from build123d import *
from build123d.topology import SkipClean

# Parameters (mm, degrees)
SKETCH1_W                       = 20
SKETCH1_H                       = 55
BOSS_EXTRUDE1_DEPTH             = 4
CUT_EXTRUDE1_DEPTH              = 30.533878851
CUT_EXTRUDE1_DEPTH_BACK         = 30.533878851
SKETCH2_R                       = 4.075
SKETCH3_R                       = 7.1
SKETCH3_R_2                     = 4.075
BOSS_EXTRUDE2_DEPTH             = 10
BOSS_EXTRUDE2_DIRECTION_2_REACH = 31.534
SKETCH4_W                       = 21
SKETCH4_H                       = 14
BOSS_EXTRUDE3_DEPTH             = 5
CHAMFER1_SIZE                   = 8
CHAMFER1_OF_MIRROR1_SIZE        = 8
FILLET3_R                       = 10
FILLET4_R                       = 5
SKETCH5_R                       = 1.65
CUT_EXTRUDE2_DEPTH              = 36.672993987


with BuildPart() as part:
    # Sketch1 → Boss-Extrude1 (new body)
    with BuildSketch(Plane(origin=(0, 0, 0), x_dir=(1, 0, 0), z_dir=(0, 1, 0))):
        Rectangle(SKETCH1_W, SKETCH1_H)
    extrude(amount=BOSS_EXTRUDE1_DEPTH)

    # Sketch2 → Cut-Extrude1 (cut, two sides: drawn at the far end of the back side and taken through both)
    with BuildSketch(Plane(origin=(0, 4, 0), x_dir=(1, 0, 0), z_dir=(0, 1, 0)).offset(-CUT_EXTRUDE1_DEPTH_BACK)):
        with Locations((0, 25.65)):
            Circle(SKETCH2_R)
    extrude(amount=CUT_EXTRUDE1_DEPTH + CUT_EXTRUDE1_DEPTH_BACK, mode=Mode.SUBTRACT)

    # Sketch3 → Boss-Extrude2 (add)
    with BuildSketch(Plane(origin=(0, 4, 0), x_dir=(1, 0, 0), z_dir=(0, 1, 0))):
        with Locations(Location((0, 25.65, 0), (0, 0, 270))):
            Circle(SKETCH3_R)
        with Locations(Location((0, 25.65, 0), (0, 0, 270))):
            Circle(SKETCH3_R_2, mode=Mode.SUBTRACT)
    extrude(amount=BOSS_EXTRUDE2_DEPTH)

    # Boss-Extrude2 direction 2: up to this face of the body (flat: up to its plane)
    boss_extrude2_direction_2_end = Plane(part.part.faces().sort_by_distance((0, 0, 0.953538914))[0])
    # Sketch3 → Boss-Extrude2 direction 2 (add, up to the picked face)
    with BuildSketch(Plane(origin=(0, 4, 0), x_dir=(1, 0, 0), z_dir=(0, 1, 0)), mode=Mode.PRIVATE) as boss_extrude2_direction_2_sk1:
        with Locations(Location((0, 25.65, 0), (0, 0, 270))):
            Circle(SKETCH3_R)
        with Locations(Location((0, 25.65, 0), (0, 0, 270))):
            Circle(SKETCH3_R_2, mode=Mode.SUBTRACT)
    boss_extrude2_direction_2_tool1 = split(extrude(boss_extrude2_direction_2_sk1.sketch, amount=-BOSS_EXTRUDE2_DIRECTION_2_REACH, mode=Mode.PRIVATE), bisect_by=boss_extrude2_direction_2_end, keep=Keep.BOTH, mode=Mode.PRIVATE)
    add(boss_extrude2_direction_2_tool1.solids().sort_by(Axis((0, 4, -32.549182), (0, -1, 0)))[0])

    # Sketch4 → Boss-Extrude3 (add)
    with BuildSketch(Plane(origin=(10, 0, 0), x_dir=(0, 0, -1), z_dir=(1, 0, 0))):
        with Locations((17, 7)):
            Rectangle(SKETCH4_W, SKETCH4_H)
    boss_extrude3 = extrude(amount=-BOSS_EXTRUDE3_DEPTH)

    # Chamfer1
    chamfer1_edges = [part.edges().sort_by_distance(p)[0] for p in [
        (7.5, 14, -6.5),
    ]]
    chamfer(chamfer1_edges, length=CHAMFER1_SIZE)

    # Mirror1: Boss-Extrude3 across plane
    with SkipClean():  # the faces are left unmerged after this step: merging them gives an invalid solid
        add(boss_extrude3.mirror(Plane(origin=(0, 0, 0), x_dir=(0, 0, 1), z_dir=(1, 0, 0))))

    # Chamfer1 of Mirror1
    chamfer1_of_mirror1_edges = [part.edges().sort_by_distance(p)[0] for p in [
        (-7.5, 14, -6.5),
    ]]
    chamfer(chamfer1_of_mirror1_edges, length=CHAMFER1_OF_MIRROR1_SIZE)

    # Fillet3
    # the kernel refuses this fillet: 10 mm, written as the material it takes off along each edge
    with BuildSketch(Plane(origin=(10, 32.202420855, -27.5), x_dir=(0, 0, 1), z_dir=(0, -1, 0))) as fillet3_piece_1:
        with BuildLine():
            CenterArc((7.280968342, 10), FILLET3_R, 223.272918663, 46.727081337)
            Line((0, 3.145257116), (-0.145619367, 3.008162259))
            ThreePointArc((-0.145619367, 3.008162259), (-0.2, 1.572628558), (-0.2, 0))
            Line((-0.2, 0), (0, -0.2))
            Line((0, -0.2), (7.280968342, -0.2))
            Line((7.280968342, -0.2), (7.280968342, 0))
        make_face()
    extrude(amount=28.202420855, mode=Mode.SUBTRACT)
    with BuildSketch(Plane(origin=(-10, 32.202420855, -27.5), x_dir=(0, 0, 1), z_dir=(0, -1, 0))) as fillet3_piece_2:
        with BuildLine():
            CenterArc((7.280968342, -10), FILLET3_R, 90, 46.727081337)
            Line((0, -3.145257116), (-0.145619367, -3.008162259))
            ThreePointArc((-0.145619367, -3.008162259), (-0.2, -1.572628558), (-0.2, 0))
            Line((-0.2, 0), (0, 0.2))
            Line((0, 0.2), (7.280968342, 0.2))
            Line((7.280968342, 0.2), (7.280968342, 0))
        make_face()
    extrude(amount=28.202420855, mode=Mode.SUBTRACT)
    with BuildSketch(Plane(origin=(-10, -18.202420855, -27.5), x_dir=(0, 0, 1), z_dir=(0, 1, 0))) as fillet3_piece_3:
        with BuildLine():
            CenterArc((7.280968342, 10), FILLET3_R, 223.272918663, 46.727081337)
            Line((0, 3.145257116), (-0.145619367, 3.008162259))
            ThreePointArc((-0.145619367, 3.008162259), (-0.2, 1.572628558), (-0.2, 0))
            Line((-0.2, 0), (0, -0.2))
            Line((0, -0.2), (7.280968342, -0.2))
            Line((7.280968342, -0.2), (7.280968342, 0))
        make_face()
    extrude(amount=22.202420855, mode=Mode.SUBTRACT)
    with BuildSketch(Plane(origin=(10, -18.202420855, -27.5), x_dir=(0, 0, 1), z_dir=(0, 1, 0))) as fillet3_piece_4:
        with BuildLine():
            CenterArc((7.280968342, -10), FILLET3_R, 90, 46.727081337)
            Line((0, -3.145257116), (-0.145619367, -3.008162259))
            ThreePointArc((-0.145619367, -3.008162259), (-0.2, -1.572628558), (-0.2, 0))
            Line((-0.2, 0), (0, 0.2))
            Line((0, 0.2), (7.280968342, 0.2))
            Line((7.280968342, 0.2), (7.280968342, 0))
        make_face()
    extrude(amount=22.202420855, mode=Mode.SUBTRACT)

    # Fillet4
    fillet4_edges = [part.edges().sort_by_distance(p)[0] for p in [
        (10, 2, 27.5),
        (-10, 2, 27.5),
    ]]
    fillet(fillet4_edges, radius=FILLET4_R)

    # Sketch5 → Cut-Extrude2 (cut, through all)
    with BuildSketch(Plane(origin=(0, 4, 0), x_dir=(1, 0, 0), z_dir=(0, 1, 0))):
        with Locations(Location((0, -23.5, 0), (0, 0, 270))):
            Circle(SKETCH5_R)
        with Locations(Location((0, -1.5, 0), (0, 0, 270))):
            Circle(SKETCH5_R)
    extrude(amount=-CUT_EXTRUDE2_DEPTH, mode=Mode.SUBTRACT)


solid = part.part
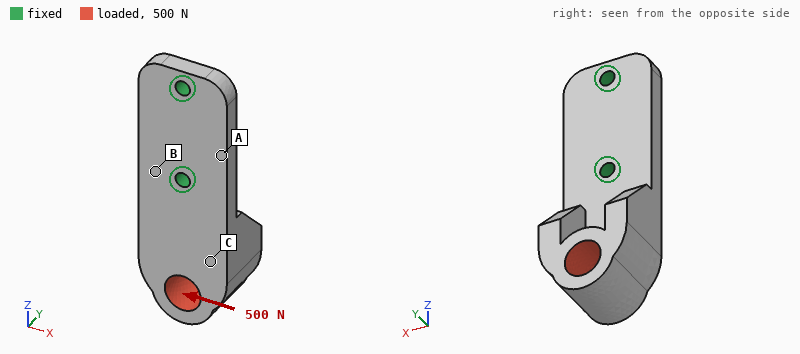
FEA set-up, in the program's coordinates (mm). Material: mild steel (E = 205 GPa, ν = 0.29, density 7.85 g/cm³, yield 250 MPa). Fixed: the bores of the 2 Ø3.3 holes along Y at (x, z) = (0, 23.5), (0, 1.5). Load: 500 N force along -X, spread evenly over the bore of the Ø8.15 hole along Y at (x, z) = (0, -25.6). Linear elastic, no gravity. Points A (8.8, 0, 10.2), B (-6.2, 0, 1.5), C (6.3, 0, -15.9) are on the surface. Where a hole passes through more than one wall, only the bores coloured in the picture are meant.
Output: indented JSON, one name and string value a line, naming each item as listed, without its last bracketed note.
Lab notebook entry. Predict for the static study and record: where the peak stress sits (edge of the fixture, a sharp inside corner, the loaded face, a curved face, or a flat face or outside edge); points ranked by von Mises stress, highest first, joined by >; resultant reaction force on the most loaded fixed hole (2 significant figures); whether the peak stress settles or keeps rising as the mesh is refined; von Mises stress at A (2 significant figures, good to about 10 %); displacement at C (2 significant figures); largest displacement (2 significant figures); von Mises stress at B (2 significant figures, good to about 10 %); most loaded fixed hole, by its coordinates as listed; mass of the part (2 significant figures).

{
  "where the peak stress sits": "edge of the fixture",
  "points ranked by von Mises stress, highest first, joined by >": "B > A > C",
  "resultant reaction force on the most loaded fixed hole": "980 N",
  "whether the peak stress settles or keeps rising as the mesh is refined": "keeps rising",
  "von Mises stress at A": "28 MPa",
  "displacement at C": "8.9 µm",
  "largest displacement": "27 µm",
  "von Mises stress at B": "43 MPa",
  "most loaded fixed hole, by its coordinates as listed": "(0, 1.5)",
  "mass of the part": "53 g"
}
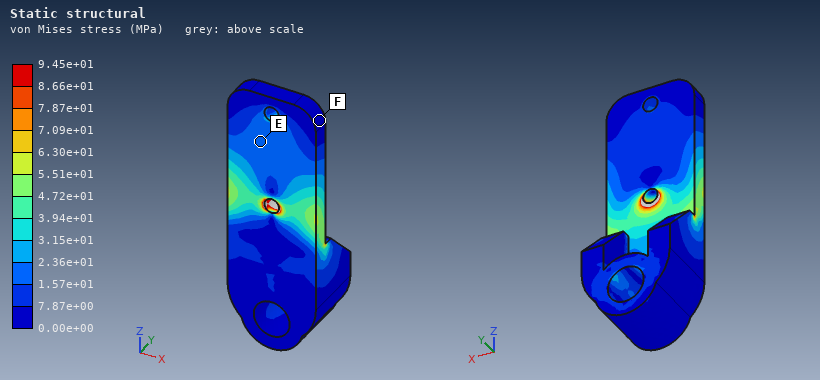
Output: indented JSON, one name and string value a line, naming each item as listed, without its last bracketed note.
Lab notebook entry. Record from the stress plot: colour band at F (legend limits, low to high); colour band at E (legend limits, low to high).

{
  "colour band at F": "0.00e+00 to 7.87e+00 MPa",
  "colour band at E": "1.57e+01 to 2.36e+01 MPa"
}
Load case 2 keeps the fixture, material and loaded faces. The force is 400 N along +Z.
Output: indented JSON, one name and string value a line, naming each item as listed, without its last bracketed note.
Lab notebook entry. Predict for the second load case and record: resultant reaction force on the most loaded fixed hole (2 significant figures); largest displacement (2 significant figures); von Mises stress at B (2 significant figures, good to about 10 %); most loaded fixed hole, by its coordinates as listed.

{
  "resultant reaction force on the most loaded fixed hole": "330 N",
  "largest displacement": "33 µm",
  "von Mises stress at B": "16 MPa",
  "most loaded fixed hole, by its coordinates as listed": "(0, 1.5)"
}
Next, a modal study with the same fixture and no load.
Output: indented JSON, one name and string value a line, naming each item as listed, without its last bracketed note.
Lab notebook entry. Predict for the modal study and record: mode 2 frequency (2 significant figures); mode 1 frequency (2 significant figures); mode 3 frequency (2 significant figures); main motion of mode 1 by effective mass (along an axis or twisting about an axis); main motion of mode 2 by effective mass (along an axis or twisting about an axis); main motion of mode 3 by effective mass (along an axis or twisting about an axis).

{
  "mode 2 frequency": "5100 Hz",
  "mode 1 frequency": "2100 Hz",
  "mode 3 frequency": "8000 Hz",
  "main motion of mode 1 by effective mass": "along Y",
  "main motion of mode 2 by effective mass": "along X",
  "main motion of mode 3 by effective mass": "along X"
}
